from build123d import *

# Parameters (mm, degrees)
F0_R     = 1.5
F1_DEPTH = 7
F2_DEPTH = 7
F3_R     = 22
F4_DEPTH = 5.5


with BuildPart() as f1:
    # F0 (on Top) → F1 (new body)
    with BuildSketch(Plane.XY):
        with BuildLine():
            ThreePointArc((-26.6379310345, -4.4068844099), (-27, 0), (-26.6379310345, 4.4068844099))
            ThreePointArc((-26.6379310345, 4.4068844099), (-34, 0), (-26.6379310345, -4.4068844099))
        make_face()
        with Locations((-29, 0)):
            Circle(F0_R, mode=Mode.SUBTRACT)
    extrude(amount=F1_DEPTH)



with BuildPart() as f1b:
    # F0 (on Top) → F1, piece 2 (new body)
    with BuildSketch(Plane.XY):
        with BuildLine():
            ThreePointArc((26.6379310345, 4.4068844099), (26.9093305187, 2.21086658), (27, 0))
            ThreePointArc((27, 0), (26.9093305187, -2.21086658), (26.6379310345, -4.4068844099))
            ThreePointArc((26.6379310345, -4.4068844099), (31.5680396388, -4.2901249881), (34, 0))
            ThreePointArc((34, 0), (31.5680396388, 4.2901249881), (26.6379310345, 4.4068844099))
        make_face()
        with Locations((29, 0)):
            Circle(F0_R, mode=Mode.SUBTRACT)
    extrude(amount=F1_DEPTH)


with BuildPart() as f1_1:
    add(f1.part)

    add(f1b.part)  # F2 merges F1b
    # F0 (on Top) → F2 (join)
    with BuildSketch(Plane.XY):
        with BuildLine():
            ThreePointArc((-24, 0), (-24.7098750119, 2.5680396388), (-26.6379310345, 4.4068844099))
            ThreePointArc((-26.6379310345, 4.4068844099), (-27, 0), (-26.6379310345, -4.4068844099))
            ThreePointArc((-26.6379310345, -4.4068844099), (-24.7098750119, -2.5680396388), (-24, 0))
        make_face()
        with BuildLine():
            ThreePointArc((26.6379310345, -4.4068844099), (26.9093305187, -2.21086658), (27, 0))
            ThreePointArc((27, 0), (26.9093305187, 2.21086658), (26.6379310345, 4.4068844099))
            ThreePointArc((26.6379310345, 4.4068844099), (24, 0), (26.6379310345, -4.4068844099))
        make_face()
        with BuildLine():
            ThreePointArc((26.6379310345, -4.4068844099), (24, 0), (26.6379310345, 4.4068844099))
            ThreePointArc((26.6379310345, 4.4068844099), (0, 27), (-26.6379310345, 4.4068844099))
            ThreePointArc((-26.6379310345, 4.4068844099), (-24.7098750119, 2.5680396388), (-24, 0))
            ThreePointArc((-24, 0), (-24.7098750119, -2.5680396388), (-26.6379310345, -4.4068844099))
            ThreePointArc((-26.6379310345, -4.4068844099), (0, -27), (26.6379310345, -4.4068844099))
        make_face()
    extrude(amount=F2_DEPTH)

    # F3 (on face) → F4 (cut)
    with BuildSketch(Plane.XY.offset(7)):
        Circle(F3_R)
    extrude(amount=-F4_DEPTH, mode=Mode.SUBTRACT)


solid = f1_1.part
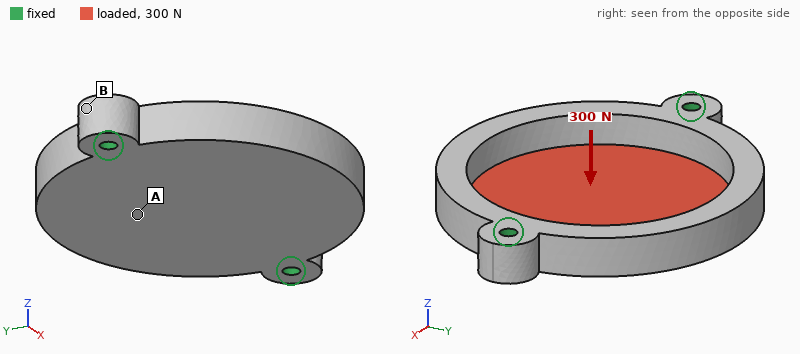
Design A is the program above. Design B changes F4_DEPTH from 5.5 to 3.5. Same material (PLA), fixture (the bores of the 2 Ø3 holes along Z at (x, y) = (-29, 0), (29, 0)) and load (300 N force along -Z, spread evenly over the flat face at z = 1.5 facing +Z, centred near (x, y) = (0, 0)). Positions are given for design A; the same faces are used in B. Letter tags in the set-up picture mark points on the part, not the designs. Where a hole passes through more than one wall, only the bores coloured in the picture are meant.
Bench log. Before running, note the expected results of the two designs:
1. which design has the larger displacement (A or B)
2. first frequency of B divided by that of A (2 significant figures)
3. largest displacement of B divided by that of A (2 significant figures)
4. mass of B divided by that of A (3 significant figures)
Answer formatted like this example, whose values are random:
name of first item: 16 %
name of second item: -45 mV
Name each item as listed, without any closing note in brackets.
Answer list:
which design has the larger displacement: A
first frequency of B divided by that of A: 0.94
largest displacement of B divided by that of A: 0.31
mass of B divided by that of A: 1.36
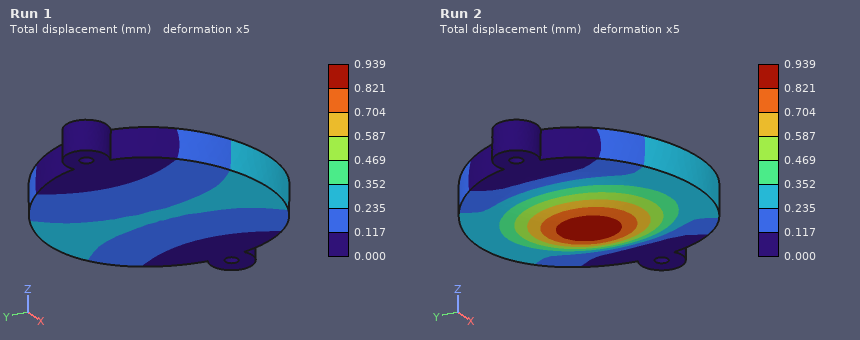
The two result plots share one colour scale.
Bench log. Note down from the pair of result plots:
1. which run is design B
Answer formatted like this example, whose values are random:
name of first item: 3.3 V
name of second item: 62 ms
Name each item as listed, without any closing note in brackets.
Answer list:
which run is design B: Run 1
